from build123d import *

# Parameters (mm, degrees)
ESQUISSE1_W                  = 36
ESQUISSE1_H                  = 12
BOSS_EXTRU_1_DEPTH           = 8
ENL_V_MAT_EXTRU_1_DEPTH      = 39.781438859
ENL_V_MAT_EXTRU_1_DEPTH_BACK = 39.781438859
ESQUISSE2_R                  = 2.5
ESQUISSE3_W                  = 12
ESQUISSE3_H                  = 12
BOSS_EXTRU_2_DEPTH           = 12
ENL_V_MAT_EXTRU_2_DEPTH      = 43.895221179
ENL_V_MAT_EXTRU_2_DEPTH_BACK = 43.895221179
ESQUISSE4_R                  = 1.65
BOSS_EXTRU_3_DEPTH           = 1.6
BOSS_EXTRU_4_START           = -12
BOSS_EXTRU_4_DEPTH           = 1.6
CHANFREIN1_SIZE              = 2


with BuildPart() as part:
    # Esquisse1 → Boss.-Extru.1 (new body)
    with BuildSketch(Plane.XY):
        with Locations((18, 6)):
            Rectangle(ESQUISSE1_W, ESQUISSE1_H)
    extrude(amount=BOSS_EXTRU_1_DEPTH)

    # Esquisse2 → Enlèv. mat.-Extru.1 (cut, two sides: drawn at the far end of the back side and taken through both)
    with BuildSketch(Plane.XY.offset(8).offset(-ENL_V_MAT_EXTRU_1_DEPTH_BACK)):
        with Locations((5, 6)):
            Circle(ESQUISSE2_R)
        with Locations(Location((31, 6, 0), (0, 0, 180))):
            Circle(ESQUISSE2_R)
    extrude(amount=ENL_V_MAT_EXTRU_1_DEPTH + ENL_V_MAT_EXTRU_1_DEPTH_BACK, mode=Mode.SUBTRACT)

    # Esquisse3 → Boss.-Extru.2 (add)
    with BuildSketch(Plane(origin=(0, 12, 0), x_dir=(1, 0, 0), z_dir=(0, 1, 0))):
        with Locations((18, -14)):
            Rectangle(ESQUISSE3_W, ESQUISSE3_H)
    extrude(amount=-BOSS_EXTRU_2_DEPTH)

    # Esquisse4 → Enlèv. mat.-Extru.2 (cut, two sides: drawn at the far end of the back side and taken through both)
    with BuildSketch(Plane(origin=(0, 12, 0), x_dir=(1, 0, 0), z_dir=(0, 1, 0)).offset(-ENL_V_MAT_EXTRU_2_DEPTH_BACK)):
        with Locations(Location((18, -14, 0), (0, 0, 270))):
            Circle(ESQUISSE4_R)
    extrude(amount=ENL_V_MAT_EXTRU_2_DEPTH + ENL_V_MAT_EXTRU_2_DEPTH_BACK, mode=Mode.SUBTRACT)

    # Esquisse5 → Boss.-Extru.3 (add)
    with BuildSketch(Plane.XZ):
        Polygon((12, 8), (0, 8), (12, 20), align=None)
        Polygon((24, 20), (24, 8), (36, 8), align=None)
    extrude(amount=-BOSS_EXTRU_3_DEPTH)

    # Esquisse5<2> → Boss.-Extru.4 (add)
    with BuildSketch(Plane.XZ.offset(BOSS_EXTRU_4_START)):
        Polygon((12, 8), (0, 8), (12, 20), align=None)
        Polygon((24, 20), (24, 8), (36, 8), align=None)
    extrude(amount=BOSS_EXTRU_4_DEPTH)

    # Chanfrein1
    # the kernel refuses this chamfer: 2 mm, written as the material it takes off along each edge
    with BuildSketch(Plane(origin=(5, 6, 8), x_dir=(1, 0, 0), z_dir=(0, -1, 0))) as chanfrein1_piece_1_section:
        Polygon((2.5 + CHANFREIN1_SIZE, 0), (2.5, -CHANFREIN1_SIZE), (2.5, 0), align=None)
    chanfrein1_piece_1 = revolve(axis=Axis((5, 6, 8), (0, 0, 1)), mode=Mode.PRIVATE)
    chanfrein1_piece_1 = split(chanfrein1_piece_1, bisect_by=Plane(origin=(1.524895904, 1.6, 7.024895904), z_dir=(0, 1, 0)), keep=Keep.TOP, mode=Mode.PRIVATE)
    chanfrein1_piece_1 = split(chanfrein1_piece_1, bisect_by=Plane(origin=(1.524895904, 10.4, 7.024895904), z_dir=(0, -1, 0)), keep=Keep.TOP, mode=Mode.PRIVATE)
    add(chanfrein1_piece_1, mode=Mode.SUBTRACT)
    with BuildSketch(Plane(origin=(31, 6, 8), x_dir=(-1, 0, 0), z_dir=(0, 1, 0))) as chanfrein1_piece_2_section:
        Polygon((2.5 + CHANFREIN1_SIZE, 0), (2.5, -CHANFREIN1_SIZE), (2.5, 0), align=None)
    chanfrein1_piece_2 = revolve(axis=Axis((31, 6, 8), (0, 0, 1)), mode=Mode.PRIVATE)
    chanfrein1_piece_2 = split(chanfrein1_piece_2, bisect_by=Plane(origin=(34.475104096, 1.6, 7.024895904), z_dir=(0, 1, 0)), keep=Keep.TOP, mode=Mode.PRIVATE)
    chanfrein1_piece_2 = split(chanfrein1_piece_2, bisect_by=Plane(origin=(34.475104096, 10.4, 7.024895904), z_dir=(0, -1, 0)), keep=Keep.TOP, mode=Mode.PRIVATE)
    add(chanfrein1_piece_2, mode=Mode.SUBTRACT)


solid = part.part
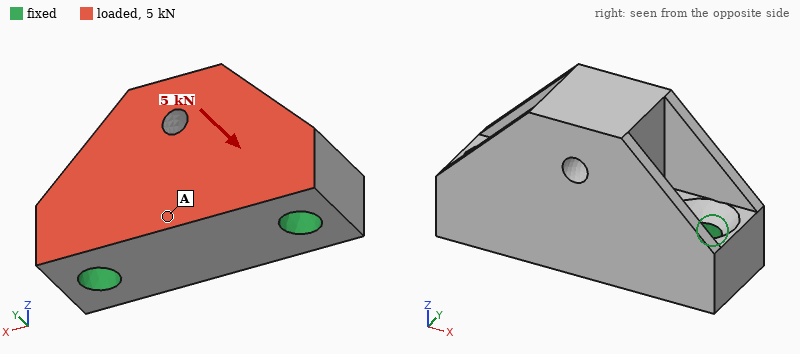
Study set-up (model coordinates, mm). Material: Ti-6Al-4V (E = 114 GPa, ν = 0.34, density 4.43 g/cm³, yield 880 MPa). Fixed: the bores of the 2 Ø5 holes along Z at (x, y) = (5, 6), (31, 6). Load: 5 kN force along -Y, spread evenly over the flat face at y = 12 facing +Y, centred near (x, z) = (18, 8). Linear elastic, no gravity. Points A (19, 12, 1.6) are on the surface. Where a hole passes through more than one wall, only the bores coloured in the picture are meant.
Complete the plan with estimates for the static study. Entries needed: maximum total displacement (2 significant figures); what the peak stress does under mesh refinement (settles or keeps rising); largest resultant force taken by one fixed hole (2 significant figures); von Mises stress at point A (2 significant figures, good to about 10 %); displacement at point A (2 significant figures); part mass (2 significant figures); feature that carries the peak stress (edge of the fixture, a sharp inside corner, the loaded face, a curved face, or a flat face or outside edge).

41 µm
keeps rising
2.5 kN
40 MPa
8.9 µm
23 g
edge of the fixture
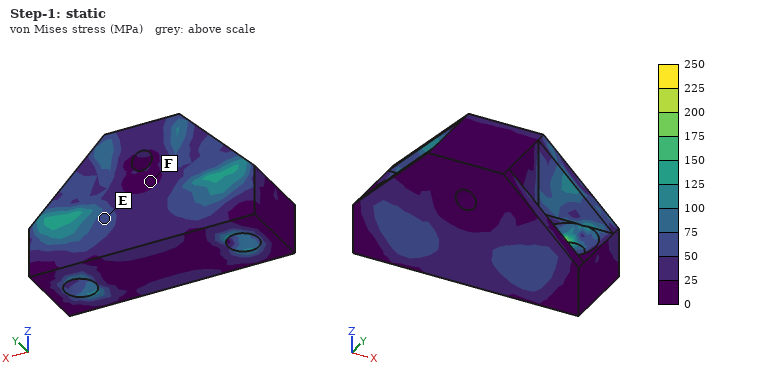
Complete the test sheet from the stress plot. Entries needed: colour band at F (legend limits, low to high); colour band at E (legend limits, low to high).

0 to 25 MPa
50 to 75 MPa
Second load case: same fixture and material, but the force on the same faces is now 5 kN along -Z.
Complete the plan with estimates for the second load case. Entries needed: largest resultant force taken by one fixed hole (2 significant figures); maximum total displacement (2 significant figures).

2.6 kN
29 µm
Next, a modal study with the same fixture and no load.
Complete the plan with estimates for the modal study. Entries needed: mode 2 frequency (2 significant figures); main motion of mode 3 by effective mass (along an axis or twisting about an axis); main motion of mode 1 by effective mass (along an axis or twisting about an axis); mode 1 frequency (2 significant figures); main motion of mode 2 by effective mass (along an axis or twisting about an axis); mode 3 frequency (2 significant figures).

36 kHz
along X
along Y
16 kHz
along Z
38 kHz
